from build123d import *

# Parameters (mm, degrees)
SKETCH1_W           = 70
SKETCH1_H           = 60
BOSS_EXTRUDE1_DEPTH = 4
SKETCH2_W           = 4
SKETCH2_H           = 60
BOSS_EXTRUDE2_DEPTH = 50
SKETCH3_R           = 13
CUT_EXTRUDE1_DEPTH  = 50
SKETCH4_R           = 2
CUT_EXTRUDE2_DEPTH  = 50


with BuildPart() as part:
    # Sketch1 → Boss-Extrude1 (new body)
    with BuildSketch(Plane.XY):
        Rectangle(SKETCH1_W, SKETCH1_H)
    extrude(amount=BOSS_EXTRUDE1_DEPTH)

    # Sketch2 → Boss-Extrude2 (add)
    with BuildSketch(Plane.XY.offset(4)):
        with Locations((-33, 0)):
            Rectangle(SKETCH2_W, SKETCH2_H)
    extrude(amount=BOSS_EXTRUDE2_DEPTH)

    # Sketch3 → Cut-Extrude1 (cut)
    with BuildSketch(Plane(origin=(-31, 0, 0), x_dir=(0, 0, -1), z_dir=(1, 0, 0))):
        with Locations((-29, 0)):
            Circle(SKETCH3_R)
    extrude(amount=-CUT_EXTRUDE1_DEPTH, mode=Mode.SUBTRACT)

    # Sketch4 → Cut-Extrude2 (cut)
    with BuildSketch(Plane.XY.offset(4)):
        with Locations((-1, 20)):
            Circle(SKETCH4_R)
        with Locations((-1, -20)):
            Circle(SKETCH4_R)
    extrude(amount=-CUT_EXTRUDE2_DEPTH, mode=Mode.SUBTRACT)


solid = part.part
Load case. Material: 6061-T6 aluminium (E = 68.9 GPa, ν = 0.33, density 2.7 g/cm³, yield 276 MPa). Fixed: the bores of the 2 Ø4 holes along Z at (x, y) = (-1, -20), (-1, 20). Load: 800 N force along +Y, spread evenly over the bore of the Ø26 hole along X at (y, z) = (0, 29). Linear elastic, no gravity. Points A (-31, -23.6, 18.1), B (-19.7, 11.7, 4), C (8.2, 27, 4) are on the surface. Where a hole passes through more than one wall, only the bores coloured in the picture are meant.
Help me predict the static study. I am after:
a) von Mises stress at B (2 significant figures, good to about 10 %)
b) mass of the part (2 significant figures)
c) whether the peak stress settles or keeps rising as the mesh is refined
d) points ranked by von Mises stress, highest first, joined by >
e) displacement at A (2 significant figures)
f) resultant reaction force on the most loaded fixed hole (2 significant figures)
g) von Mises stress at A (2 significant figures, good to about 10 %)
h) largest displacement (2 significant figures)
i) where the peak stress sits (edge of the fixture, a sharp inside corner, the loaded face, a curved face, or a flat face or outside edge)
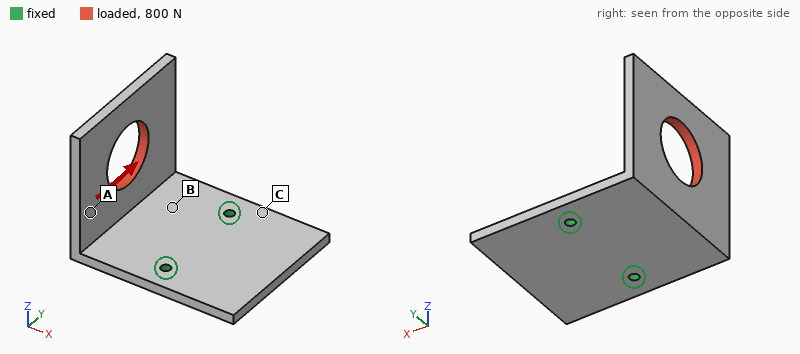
73 MPa
72 g
keeps rising
B > A > C
0.27 mm
880 N
31 MPa
0.59 mm
edge of the fixture
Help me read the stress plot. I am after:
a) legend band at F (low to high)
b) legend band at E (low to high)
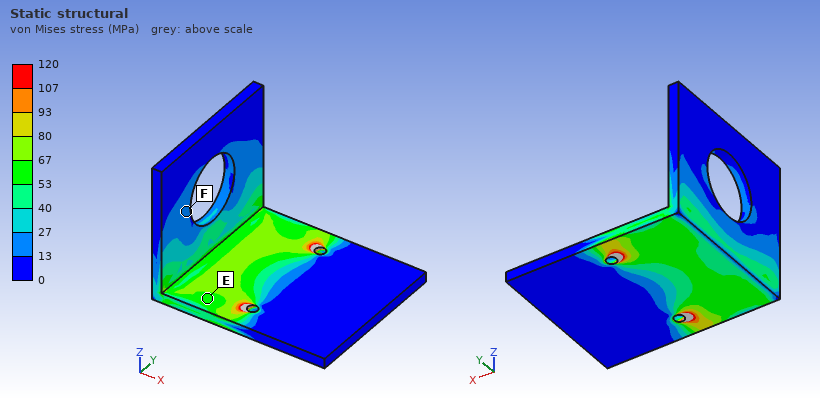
13 to 27 MPa
53 to 67 MPa
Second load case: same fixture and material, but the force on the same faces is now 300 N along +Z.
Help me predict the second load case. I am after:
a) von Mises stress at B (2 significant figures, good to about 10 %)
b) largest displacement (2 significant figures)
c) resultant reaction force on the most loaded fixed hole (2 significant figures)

22 MPa
0.42 mm
150 N
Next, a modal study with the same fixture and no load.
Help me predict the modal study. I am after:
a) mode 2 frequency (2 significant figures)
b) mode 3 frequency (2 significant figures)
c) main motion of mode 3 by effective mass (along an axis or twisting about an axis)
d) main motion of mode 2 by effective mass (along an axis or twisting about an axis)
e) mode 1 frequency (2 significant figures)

1200 Hz
1700 Hz
along Z
along Y
620 Hz
